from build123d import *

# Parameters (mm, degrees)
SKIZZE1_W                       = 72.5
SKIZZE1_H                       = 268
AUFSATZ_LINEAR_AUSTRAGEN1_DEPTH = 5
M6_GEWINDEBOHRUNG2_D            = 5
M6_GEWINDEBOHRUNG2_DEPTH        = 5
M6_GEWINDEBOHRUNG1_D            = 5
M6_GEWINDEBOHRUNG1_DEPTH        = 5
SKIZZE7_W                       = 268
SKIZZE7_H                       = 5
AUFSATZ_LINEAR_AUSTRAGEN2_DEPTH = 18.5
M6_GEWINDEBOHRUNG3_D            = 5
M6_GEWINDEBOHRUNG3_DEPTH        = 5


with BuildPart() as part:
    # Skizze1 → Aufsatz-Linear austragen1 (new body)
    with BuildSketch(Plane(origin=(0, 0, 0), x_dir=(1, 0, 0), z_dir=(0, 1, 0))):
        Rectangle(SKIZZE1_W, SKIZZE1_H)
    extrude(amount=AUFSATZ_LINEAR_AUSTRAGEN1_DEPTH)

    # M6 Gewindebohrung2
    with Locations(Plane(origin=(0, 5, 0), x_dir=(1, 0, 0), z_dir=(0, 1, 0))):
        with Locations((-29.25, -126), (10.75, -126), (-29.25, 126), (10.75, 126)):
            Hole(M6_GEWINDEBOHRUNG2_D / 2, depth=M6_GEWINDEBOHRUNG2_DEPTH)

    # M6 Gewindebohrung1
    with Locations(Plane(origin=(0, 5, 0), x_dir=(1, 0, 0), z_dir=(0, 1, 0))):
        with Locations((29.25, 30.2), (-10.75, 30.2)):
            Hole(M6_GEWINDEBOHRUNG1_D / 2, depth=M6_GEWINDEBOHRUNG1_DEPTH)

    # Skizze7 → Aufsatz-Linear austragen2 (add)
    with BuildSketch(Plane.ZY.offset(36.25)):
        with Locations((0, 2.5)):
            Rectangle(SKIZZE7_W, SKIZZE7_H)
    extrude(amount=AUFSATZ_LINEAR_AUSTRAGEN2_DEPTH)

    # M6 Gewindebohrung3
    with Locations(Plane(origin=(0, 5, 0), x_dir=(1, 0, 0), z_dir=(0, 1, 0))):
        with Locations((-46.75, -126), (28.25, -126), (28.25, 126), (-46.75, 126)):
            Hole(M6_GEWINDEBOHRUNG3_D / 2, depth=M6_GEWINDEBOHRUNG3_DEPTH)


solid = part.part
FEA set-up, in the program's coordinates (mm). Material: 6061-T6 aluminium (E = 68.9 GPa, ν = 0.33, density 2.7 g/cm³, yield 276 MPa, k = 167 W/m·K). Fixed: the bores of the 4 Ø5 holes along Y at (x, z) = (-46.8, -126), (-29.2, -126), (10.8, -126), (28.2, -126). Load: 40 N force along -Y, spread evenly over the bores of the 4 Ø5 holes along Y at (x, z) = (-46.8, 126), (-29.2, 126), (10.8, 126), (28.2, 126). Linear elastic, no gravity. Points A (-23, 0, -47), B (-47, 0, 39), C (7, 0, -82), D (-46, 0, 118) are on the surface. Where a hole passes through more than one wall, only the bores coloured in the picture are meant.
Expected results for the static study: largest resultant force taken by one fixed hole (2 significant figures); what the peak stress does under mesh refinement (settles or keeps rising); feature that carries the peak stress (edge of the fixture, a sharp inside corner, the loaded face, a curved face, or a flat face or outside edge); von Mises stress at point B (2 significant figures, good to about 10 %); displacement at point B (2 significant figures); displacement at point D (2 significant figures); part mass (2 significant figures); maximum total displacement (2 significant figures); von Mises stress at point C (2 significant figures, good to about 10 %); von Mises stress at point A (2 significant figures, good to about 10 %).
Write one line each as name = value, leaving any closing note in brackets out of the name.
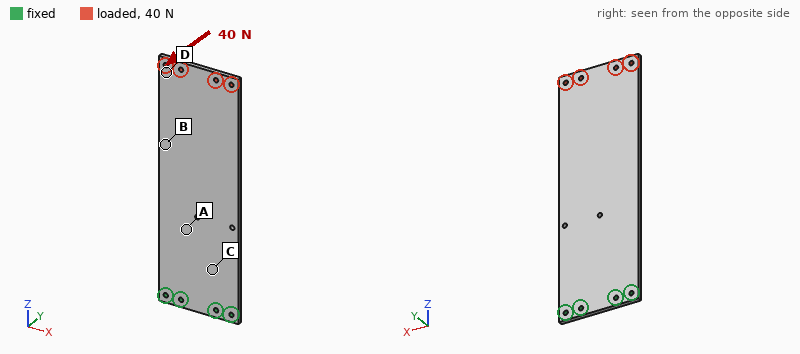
largest resultant force taken by one fixed hole = 60 N
what the peak stress does under mesh refinement = keeps rising
feature that carries the peak stress = edge of the fixture
von Mises stress at point B = 9.4 MPa
displacement at point B = 1.6 mm
displacement at point D = 3.1 mm
part mass = 330 g
maximum total displacement = 3.4 mm
von Mises stress at point C = 20 MPa
von Mises stress at point A = 18 MPa
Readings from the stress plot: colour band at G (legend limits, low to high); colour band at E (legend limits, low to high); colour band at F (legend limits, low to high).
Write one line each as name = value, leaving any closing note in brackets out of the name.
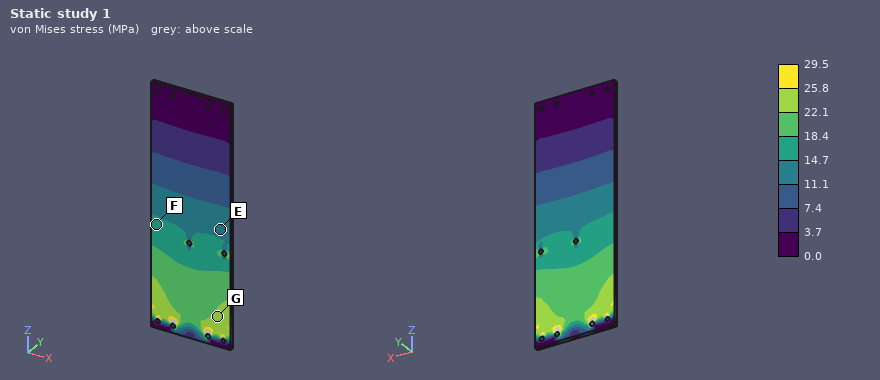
colour band at G = 22.1 to 25.8 MPa
colour band at E = 11.1 to 14.7 MPa
colour band at F = 14.7 to 18.4 MPa
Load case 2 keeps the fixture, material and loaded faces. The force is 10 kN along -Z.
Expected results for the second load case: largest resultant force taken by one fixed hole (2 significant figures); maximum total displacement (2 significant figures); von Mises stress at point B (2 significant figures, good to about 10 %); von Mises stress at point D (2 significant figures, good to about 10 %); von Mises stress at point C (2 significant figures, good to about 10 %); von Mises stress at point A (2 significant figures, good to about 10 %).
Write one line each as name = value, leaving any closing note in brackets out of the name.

largest resultant force taken by one fixed hole = 2.8 kN
maximum total displacement = 90 µm
von Mises stress at point B = 22 MPa
von Mises stress at point D = 32 MPa
von Mises stress at point C = 21 MPa
von Mises stress at point A = 22 MPa
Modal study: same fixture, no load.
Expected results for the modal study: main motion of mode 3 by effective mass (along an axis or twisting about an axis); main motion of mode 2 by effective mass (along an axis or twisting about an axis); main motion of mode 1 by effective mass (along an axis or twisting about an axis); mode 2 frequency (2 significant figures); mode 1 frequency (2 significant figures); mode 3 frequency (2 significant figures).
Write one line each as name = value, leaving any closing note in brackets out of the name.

main motion of mode 3 by effective mass = along Y
main motion of mode 2 by effective mass = twisting about Z
main motion of mode 1 by effective mass = along Y
mode 2 frequency = 360 Hz
mode 1 frequency = 61 Hz
mode 3 frequency = 380 Hz
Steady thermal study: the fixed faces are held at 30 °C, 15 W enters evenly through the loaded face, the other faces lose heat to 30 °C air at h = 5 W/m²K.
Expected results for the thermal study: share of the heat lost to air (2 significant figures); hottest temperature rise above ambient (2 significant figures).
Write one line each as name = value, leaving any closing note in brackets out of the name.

share of the heat lost to air = 32 %
hottest temperature rise above ambient = 41 K
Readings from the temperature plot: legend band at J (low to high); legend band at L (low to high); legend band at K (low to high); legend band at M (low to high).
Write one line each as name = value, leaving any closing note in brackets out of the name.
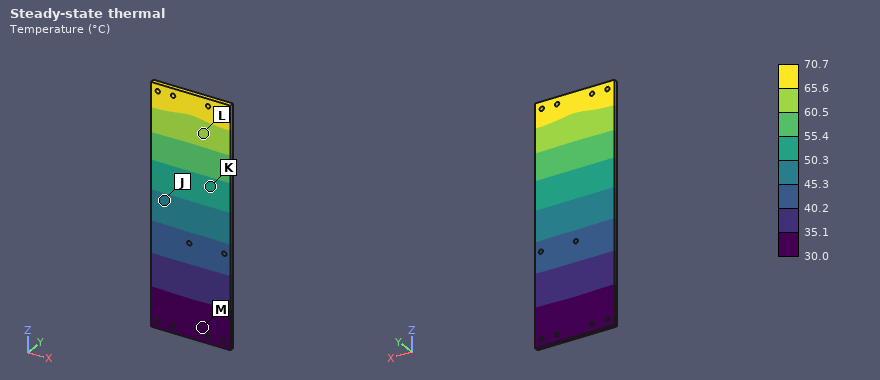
legend band at J = 45.3 to 50.3 °C
legend band at L = 60.5 to 65.6 °C
legend band at K = 50.3 to 55.4 °C
legend band at M = 30.0 to 35.1 °C
